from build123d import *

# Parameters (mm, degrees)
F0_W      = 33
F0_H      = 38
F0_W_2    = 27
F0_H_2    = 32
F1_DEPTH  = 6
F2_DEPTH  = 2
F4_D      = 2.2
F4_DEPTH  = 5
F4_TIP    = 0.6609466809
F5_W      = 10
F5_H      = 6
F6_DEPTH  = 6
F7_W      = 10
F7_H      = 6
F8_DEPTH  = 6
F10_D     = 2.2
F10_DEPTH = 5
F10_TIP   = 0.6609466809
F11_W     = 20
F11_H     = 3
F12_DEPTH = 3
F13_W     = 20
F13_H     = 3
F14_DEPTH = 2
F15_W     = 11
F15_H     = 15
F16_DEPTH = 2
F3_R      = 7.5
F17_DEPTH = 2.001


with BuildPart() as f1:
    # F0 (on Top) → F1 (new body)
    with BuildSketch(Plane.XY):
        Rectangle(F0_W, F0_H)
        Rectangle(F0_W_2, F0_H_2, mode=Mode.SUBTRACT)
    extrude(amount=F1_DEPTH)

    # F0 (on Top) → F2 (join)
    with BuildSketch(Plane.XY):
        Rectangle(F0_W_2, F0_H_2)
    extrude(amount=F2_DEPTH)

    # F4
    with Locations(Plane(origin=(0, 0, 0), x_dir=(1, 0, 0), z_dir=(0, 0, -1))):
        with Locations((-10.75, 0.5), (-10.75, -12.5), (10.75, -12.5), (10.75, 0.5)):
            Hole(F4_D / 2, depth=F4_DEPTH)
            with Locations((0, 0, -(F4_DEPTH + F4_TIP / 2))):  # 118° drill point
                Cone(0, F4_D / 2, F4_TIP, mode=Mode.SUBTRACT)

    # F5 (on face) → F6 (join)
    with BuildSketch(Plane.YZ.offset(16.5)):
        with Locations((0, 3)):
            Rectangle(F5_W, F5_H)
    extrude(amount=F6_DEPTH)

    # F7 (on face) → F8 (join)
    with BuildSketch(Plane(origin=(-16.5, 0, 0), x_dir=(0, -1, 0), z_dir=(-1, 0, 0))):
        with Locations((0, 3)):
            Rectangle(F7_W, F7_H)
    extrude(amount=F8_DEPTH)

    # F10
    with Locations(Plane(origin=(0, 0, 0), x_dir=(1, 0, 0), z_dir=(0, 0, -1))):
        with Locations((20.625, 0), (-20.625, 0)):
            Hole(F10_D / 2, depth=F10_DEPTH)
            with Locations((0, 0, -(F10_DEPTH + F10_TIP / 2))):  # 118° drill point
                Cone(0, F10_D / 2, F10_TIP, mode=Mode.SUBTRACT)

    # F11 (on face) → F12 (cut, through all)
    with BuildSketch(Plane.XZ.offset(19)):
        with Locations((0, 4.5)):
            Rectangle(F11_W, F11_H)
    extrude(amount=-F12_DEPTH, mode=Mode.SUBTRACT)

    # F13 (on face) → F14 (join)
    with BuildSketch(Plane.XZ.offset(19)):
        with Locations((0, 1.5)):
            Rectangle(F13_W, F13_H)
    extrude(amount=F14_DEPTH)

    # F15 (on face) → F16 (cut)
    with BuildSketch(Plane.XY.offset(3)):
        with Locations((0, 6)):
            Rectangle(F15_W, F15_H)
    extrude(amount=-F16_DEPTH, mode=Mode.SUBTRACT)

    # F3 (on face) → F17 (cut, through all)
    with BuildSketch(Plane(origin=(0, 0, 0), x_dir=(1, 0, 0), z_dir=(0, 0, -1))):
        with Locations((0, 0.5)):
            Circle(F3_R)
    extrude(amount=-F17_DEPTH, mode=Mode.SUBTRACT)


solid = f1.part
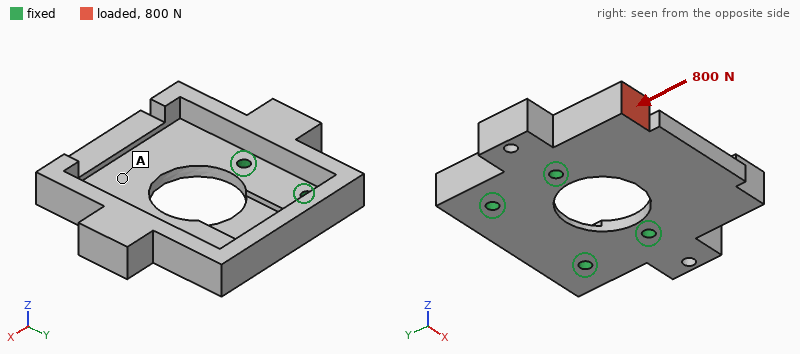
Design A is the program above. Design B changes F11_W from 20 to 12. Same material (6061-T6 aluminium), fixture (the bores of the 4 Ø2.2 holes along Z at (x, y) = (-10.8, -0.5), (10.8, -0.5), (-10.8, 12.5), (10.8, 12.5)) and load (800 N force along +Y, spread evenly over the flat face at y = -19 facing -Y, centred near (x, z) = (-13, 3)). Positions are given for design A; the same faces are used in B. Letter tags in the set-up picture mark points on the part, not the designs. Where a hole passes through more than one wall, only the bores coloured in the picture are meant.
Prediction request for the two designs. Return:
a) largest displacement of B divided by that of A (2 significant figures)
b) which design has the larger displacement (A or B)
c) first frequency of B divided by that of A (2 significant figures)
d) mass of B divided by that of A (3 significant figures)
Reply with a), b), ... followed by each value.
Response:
a) 1.3
b) B
c) 0.96
d) 1.02
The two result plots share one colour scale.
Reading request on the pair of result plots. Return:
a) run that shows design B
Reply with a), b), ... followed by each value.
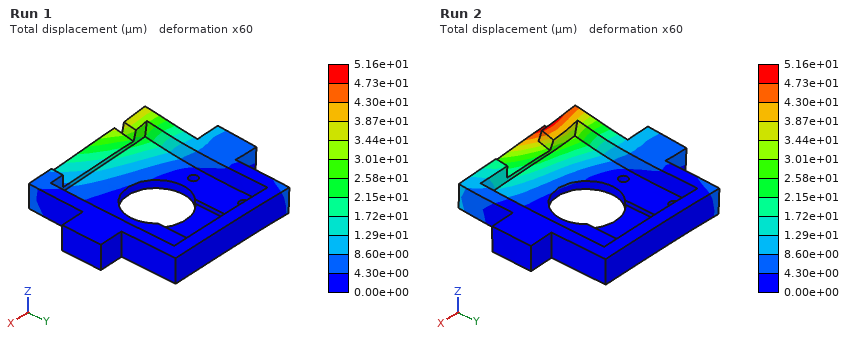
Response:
a) Run 2
